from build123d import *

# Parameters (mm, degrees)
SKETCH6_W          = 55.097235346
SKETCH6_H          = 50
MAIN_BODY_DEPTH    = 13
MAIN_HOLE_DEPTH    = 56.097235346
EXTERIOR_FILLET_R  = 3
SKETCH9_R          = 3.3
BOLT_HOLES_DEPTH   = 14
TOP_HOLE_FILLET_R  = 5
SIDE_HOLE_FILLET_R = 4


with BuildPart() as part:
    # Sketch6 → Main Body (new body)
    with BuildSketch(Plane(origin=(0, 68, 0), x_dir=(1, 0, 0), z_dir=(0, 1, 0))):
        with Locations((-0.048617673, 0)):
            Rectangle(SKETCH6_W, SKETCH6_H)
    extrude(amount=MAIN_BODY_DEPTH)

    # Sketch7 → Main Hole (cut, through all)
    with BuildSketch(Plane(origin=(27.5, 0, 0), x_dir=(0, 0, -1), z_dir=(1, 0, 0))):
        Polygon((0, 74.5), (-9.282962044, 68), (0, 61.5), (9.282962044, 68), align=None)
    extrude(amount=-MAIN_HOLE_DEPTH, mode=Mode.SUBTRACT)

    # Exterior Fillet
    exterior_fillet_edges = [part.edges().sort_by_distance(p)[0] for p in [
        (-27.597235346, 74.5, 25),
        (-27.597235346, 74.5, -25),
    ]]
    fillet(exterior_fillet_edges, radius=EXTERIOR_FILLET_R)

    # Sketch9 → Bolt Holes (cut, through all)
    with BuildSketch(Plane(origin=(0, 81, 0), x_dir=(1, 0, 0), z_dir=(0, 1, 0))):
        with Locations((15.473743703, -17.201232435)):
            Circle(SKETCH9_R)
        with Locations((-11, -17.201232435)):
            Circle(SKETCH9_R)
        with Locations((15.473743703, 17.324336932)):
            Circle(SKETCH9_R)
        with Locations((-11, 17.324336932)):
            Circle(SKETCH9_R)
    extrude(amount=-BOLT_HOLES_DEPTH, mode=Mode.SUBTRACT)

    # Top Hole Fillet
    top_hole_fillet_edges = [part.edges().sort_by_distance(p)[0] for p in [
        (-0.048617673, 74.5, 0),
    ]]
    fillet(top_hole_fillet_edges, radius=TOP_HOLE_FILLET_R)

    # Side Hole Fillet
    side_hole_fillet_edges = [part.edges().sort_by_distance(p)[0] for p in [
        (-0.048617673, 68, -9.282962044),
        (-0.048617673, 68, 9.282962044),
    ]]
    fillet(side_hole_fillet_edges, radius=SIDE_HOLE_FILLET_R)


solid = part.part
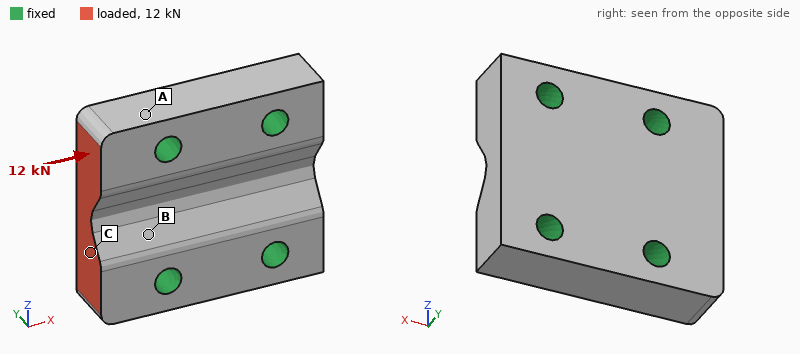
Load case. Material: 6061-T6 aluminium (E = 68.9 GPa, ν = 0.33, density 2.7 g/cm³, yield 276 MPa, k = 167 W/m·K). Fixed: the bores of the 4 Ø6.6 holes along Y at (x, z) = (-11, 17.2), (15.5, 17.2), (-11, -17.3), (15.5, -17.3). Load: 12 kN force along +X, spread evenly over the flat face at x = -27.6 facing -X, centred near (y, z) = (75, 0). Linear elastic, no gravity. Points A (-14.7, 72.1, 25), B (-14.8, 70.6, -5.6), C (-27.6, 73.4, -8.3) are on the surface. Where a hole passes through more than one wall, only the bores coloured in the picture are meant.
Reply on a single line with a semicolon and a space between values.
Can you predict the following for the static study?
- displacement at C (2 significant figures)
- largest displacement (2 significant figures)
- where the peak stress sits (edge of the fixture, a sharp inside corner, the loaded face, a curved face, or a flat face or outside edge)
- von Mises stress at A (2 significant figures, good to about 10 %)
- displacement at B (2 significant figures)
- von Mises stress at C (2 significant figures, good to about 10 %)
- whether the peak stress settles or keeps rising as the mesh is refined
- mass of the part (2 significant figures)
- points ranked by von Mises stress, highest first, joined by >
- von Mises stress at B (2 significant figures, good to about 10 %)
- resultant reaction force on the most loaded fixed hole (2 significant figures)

7.0 µm; 9.1 µm; edge of the fixture; 5.6 MPa; 3.7 µm; 22 MPa; keeps rising; 83 g; C > B > A; 14 MPa; 5.3 kN
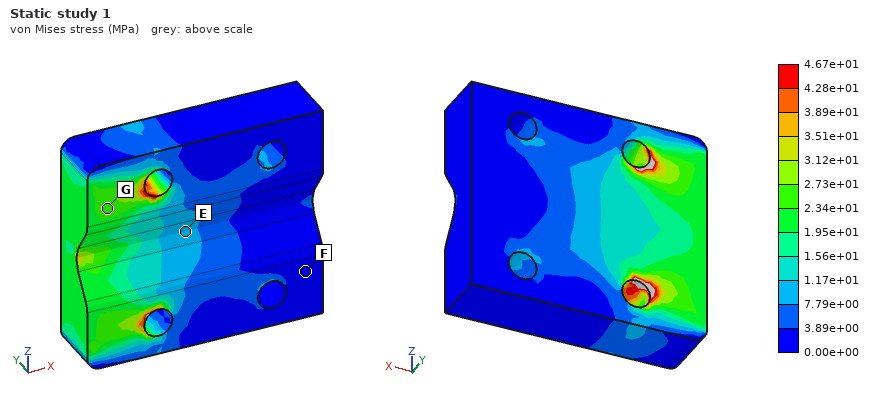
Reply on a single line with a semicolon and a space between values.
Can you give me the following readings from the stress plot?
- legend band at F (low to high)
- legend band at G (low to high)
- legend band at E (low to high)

0.00e+00 to 3.89e+00 MPa; 2.34e+01 to 2.73e+01 MPa; 7.79e+00 to 1.17e+01 MPa
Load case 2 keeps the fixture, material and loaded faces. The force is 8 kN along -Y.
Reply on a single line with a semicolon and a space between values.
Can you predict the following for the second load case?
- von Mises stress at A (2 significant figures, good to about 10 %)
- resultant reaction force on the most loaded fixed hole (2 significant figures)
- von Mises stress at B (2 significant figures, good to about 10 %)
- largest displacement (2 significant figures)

21 MPa; 4.5 kN; 42 MPa; 46 µm
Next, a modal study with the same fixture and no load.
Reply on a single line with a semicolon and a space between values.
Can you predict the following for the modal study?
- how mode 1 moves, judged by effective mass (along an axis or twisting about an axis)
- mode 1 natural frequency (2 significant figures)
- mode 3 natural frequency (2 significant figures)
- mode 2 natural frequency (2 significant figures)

along Y; 26 kHz; 34 kHz; 34 kHz
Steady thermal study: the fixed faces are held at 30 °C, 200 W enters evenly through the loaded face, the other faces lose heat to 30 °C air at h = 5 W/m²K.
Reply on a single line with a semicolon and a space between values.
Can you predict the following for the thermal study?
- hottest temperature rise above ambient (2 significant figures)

39 K
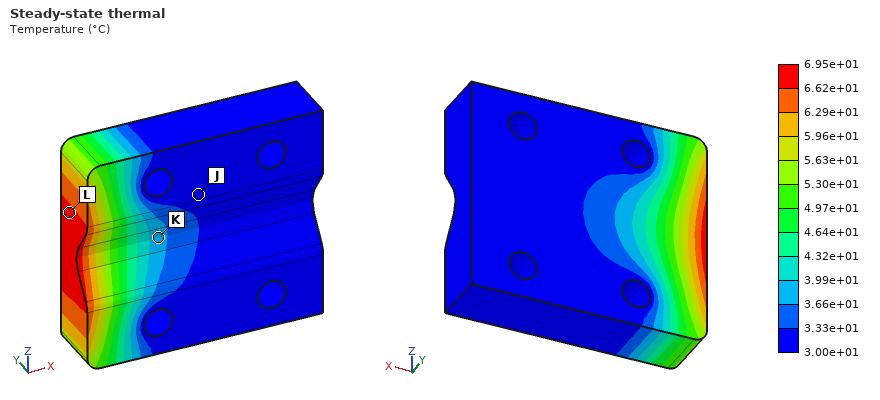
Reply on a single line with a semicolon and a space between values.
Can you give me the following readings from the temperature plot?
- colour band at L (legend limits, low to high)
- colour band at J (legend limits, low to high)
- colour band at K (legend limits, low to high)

6.62e+01 to 6.95e+01 °C; 3.00e+01 to 3.33e+01 °C; 3.66e+01 to 3.99e+01 °C
